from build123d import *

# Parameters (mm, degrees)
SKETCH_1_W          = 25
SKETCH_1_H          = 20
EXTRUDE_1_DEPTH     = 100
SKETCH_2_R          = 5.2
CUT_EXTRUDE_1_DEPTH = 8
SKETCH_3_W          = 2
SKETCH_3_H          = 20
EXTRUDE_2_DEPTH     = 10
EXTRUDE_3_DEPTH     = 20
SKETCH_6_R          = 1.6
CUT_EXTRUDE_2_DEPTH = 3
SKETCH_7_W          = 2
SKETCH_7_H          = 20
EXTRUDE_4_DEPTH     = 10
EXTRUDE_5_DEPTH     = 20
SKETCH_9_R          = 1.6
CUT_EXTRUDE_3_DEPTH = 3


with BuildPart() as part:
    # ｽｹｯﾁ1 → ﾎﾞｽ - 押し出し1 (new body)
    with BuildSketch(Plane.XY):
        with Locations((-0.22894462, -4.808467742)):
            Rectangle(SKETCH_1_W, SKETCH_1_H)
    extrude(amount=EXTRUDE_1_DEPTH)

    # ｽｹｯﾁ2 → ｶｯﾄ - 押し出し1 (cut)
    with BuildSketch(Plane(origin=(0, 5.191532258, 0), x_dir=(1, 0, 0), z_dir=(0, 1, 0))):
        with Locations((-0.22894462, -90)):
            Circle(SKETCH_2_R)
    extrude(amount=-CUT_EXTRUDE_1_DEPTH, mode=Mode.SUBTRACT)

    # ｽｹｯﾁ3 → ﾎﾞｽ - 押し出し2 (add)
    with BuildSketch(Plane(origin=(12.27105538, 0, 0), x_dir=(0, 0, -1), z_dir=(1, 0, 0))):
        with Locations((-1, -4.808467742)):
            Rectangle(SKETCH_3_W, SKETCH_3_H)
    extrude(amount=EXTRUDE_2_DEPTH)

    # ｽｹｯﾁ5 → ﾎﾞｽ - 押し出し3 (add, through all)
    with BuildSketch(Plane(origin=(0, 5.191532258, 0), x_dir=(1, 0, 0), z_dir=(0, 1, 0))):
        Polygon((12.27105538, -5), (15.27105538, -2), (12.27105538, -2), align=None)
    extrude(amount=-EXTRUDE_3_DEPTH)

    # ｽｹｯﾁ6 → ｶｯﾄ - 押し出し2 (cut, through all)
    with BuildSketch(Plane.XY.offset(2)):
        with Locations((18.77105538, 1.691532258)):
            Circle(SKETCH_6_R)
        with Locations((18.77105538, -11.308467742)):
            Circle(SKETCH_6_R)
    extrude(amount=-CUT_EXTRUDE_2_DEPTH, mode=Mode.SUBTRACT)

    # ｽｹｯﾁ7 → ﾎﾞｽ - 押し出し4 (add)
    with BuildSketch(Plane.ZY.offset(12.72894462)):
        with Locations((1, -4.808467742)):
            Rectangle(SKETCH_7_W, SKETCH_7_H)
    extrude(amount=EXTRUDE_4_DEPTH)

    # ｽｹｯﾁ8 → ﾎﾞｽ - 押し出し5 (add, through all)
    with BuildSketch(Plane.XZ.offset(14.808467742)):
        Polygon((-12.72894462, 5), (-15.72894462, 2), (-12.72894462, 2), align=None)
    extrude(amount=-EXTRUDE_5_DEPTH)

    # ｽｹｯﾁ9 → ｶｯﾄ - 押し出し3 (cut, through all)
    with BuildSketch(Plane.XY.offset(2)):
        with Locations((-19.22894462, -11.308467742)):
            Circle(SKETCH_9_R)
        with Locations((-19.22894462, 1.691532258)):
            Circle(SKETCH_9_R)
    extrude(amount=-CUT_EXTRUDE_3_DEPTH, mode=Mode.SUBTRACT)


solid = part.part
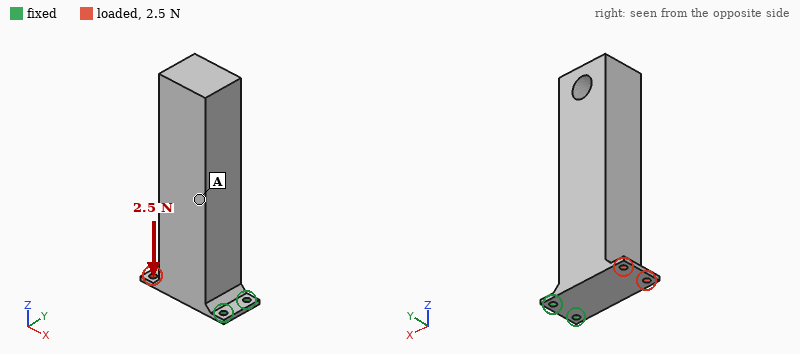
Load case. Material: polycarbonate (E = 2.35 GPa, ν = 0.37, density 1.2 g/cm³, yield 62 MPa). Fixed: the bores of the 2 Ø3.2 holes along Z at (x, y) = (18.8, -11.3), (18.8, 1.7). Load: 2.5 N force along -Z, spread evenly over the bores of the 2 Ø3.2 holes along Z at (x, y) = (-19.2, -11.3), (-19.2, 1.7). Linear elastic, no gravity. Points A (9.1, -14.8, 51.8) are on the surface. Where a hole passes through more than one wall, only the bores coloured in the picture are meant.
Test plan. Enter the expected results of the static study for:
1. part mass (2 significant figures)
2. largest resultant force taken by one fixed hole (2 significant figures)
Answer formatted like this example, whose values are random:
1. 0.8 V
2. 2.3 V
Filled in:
1. 60 g
2. 1.3 N
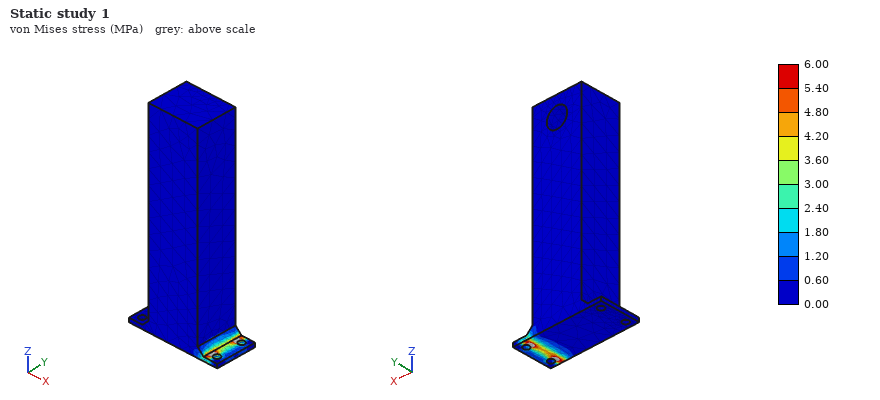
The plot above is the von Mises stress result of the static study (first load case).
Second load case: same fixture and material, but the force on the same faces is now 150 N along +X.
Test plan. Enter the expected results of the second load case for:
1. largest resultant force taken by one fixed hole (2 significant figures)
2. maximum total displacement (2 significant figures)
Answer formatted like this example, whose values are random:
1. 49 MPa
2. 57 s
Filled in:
1. 76 N
2. 0.35 mm
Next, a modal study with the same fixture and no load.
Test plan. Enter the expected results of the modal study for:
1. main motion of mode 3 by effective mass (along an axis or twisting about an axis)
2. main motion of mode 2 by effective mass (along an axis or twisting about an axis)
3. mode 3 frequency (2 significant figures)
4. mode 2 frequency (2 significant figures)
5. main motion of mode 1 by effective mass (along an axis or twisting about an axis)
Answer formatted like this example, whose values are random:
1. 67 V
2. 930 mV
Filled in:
1. along Z
2. along Y
3. 840 Hz
4. 100 Hz
5. along X
